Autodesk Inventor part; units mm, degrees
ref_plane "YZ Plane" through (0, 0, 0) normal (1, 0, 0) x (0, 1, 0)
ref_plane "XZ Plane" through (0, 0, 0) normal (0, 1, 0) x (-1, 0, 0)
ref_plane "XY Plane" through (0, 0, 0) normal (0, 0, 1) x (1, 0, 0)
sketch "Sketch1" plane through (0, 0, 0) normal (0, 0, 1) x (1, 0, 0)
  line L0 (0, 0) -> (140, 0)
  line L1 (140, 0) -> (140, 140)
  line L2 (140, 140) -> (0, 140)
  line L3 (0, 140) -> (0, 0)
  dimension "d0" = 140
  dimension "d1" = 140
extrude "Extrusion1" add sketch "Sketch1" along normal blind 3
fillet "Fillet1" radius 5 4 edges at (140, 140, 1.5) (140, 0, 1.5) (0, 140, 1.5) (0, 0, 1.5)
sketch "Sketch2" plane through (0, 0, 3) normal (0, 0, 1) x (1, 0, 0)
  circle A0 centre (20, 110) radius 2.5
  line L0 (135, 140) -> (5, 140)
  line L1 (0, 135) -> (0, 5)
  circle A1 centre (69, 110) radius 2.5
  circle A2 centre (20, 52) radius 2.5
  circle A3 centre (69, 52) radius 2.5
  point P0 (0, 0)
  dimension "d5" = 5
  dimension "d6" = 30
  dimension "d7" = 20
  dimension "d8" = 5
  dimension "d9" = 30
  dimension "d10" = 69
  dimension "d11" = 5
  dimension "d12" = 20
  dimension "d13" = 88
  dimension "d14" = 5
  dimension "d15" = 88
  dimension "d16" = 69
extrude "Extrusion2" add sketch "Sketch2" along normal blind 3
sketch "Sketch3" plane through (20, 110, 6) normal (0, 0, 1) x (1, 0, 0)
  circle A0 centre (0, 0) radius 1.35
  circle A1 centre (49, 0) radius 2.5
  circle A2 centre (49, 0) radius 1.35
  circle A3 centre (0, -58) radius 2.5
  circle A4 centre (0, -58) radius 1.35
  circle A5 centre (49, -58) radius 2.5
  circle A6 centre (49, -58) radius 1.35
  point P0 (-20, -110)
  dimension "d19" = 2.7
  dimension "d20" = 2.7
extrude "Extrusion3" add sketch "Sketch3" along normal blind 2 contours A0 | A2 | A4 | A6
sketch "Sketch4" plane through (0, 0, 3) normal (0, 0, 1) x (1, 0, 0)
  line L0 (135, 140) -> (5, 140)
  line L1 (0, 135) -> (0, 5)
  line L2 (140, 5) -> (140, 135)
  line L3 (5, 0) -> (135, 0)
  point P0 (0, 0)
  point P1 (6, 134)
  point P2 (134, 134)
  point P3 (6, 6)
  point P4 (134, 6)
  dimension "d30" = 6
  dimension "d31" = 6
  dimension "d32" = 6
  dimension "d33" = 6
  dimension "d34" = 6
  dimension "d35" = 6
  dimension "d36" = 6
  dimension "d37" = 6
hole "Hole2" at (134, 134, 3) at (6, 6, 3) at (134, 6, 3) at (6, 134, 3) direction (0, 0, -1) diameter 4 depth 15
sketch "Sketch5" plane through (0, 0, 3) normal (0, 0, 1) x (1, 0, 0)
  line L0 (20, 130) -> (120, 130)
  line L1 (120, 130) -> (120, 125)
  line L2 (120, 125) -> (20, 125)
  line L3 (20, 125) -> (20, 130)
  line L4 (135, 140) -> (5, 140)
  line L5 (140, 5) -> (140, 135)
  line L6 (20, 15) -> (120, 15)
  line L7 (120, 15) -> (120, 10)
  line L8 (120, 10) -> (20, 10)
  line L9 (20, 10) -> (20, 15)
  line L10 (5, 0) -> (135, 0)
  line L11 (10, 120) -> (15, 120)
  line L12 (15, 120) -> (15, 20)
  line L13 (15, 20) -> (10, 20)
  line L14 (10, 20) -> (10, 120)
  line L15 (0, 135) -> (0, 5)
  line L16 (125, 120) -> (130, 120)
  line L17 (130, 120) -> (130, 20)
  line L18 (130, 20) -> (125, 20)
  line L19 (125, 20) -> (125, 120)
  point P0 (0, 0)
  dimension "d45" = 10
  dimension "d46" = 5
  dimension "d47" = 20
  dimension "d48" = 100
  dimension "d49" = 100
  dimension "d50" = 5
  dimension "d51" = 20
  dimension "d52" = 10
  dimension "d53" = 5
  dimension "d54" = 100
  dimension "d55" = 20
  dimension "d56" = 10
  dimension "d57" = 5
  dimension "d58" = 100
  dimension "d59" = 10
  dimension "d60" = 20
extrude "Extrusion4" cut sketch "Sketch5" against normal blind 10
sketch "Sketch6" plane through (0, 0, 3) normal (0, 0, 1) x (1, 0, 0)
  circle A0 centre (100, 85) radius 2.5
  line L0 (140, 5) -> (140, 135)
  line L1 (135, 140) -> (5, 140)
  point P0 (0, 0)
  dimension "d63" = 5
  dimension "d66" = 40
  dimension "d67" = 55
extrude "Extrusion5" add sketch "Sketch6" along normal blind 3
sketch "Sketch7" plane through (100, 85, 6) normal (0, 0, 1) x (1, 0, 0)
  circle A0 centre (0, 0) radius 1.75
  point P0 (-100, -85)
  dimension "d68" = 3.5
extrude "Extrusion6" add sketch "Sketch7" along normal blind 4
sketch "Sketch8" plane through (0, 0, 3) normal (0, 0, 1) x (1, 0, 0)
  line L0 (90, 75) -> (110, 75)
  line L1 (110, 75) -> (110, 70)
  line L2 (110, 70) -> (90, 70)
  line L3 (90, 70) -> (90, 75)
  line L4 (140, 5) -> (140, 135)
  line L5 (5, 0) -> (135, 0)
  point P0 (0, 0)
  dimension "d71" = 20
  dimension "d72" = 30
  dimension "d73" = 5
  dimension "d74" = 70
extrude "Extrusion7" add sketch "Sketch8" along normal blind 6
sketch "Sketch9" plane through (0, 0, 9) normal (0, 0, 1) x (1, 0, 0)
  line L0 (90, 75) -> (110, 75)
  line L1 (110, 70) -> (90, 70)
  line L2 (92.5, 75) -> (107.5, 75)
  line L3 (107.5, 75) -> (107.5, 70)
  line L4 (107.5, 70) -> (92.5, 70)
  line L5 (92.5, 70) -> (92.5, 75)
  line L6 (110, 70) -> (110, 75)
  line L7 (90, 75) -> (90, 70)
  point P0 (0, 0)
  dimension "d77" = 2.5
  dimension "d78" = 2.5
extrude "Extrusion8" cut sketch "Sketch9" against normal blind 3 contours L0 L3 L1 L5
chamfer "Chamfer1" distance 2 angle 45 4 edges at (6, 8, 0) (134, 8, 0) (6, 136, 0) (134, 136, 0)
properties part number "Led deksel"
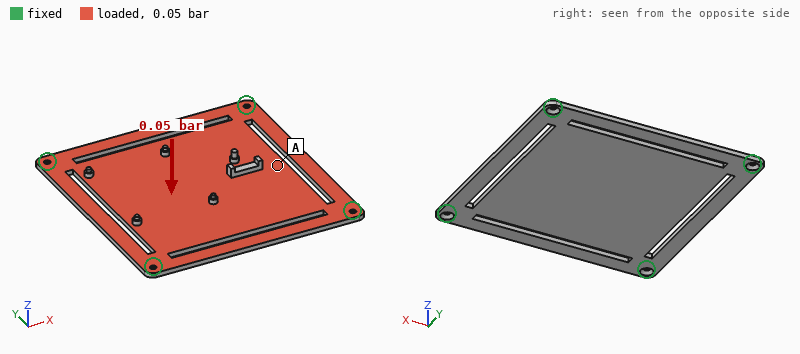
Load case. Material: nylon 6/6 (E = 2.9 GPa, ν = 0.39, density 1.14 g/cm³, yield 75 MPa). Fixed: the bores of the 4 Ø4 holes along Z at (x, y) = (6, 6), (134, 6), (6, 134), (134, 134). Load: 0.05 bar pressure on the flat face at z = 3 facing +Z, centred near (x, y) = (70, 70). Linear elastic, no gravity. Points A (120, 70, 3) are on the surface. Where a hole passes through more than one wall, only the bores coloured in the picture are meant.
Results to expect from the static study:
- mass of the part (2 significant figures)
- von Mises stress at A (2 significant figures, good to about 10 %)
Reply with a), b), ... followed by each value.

a) 61 g
b) 3.9 MPa
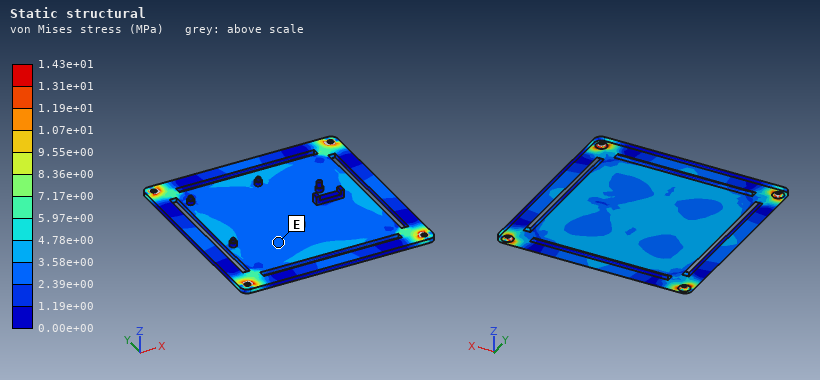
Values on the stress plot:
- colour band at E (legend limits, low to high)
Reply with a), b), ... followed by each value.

a) 2.39e+00 to 3.58e+00 MPa
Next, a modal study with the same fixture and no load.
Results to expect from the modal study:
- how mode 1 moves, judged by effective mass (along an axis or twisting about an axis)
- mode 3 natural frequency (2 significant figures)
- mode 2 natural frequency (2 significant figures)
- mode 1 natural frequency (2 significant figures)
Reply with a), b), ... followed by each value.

a) along Z
b) 280 Hz
c) 280 Hz
d) 150 Hz
